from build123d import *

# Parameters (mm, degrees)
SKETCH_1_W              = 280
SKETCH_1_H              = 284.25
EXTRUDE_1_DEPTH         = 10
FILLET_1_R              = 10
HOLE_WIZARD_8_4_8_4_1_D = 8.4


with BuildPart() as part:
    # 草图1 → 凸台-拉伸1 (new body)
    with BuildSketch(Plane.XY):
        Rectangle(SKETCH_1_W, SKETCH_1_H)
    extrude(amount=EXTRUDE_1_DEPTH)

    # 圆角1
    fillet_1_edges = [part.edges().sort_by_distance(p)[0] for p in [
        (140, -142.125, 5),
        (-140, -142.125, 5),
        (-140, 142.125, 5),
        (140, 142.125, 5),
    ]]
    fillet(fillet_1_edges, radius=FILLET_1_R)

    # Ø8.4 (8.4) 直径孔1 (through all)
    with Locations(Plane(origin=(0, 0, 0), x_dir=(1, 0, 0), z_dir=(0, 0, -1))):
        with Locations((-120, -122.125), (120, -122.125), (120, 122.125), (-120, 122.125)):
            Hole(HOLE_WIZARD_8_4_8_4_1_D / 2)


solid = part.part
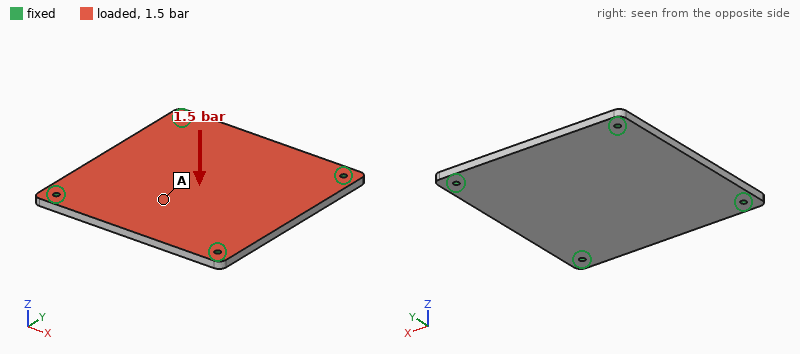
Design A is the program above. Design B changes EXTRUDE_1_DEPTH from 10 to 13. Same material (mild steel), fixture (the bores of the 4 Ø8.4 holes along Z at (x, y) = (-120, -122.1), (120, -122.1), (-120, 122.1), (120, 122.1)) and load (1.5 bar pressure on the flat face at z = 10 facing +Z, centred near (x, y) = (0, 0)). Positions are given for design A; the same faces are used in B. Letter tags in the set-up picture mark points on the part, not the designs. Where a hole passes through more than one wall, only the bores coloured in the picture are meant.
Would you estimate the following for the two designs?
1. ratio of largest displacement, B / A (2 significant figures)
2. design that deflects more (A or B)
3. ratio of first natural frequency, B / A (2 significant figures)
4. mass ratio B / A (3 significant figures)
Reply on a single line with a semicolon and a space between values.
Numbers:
0.47; A; 1.3; 1.30
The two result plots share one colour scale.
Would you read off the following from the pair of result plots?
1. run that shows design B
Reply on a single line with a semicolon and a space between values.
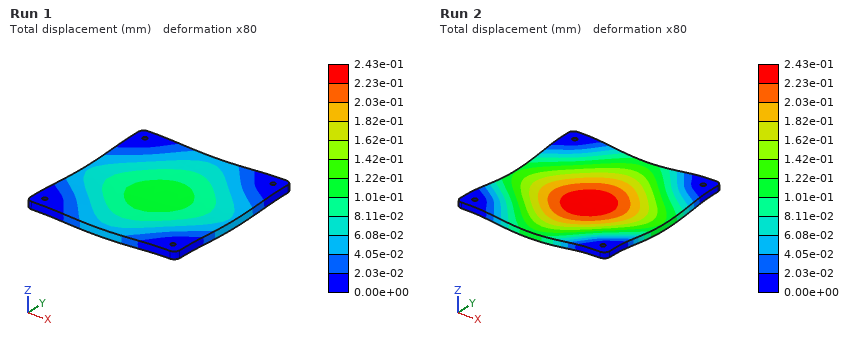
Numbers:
Run 1
